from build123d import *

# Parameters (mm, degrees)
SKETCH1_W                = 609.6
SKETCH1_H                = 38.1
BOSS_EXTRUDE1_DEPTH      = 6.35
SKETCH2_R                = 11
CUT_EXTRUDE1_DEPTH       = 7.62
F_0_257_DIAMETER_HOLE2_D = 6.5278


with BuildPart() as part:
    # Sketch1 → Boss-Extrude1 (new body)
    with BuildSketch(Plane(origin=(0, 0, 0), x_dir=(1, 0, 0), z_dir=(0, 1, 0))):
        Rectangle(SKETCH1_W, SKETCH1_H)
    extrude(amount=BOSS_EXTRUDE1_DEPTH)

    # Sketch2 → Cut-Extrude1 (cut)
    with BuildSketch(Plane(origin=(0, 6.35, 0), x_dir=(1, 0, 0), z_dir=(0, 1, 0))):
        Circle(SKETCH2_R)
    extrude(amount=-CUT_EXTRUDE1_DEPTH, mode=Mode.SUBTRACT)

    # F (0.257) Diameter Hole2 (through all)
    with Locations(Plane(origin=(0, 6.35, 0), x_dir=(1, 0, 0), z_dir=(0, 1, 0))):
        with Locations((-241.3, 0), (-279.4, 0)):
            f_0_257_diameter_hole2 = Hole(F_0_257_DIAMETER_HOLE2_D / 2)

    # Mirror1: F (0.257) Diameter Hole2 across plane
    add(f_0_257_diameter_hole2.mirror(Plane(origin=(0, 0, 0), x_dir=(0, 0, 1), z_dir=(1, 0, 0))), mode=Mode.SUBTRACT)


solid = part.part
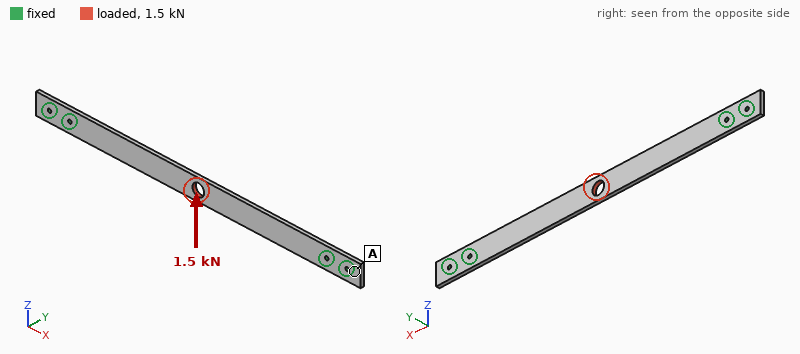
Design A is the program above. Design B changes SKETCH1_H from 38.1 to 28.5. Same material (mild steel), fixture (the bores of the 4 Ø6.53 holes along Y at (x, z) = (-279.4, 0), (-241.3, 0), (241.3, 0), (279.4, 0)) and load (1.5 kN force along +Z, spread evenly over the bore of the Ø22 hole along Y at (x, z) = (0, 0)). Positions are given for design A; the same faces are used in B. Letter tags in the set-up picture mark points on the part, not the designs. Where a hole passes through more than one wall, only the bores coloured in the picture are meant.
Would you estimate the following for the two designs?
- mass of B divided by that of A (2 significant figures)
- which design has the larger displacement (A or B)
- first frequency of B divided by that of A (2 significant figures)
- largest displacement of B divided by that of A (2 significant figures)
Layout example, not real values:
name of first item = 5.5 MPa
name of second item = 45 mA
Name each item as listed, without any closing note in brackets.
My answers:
mass of B divided by that of A = 0.74
which design has the larger displacement = B
first frequency of B divided by that of A = 0.99
largest displacement of B divided by that of A = 2.3
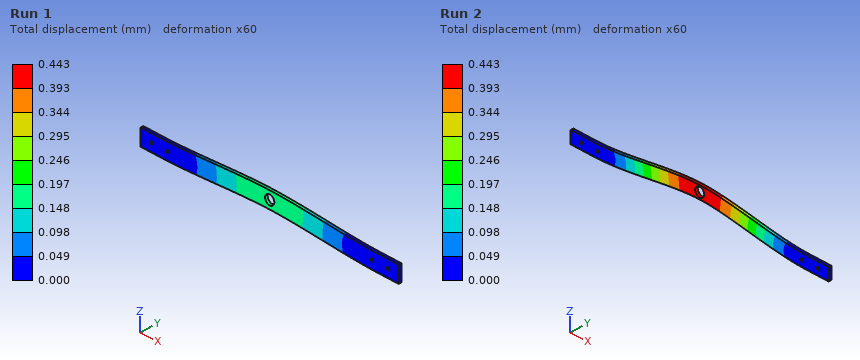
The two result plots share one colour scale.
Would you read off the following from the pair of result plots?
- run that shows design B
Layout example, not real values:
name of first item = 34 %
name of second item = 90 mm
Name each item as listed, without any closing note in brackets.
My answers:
run that shows design B = Run 2
